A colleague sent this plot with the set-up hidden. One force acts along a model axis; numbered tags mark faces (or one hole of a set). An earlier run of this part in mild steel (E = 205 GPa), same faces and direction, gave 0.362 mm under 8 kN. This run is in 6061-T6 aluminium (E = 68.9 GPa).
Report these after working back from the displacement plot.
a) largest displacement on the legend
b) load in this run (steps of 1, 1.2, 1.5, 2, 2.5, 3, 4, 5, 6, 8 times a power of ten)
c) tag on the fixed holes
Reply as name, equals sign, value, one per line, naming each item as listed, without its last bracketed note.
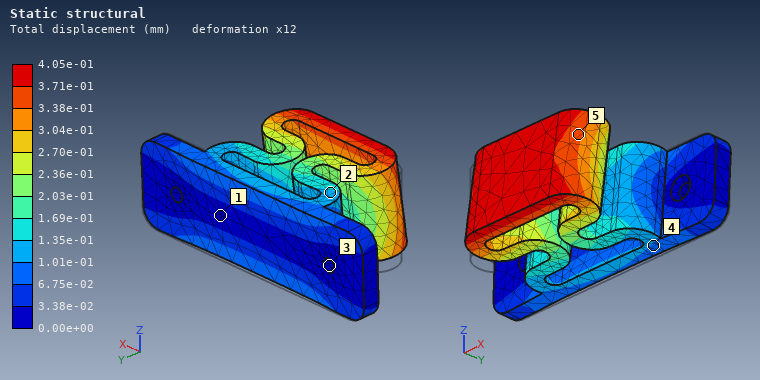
largest displacement on the legend = 4.05e-01 mm
load in this run = 3 kN
tag on the fixed holes = 3
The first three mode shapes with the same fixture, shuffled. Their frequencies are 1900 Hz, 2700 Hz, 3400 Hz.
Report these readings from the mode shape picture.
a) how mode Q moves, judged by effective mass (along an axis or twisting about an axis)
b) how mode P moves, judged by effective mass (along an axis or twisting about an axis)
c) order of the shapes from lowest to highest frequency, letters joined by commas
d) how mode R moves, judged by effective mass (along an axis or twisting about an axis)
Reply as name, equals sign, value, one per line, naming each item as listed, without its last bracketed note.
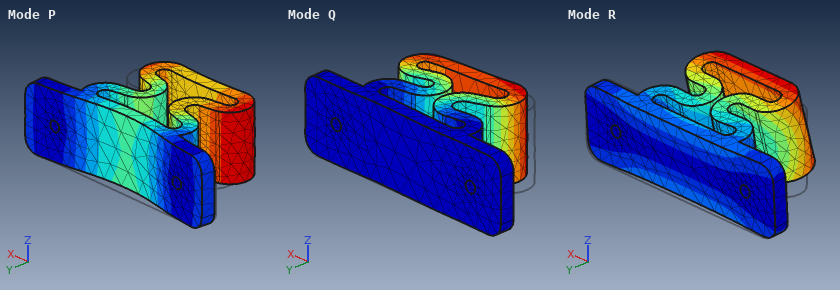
how mode Q moves, judged by effective mass = along X
how mode P moves, judged by effective mass = along Y
order of the shapes from lowest to highest frequency, letters joined by commas = R, Q, P
how mode R moves, judged by effective mass = along Z
